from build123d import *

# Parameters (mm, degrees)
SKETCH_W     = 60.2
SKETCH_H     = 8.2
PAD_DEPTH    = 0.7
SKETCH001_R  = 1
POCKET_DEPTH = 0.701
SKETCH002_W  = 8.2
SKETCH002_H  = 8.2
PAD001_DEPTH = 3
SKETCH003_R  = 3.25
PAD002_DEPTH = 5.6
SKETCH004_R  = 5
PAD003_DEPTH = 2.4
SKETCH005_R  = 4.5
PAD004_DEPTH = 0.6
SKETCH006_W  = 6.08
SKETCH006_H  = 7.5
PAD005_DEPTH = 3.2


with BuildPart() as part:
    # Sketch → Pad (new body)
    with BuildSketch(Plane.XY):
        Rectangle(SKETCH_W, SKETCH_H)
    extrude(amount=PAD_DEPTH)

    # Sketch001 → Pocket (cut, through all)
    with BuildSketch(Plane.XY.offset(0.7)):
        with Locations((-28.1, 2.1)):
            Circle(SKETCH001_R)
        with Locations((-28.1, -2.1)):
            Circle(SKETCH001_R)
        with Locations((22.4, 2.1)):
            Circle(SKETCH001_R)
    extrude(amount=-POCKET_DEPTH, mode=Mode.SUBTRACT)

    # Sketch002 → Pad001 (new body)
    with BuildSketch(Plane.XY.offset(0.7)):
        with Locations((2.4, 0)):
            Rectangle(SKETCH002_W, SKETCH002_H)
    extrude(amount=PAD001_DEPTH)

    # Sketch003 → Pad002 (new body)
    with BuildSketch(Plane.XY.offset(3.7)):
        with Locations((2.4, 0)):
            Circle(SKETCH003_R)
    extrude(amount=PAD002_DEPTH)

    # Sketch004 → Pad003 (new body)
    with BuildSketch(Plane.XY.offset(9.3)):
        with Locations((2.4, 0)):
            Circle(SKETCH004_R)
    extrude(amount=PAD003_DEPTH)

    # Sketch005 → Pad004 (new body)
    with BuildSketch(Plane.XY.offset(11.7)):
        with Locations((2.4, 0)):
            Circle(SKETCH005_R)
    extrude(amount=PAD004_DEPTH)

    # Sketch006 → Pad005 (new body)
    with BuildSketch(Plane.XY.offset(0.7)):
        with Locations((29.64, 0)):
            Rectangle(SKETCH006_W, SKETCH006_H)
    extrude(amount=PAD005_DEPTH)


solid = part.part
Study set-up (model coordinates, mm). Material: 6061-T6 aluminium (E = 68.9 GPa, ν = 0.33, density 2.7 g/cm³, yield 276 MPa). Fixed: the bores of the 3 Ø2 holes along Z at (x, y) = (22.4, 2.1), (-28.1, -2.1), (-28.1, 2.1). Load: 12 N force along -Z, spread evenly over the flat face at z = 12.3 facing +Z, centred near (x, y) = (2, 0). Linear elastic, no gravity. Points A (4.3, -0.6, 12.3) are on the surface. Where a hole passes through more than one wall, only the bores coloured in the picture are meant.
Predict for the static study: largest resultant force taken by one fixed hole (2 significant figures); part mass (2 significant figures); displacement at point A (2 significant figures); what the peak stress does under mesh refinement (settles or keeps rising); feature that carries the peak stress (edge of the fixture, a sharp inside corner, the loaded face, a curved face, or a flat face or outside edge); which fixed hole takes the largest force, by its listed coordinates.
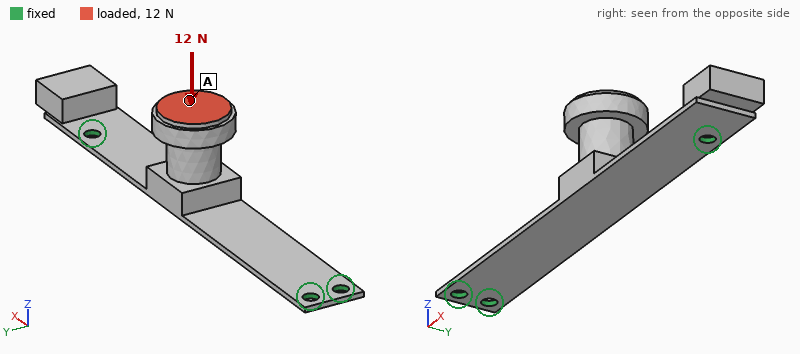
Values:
8.8 N
3.0 g
0.24 mm
keeps rising
edge of the fixture
(22.4, 2.1)
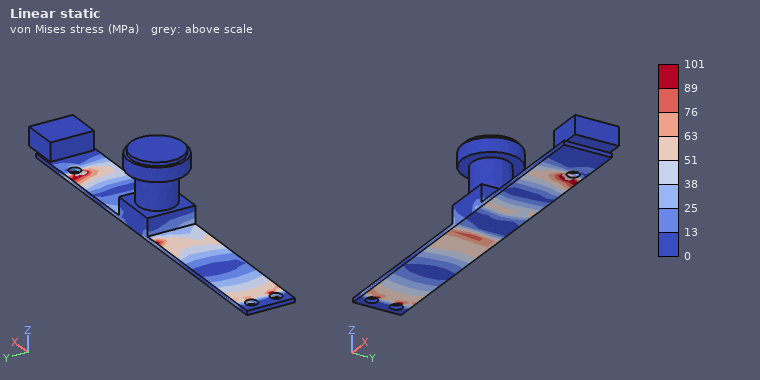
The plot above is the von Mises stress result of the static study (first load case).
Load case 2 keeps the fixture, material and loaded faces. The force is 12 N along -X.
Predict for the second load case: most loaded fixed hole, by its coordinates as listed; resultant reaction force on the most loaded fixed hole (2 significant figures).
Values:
(22.4, 2.1)
7.1 N
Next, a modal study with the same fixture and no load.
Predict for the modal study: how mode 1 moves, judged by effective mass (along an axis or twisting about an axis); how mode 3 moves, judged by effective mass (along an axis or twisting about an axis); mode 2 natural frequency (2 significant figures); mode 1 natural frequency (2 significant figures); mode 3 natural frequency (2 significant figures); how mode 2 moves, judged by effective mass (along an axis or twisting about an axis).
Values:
along Z
along X
850 Hz
760 Hz
1800 Hz
along Y
